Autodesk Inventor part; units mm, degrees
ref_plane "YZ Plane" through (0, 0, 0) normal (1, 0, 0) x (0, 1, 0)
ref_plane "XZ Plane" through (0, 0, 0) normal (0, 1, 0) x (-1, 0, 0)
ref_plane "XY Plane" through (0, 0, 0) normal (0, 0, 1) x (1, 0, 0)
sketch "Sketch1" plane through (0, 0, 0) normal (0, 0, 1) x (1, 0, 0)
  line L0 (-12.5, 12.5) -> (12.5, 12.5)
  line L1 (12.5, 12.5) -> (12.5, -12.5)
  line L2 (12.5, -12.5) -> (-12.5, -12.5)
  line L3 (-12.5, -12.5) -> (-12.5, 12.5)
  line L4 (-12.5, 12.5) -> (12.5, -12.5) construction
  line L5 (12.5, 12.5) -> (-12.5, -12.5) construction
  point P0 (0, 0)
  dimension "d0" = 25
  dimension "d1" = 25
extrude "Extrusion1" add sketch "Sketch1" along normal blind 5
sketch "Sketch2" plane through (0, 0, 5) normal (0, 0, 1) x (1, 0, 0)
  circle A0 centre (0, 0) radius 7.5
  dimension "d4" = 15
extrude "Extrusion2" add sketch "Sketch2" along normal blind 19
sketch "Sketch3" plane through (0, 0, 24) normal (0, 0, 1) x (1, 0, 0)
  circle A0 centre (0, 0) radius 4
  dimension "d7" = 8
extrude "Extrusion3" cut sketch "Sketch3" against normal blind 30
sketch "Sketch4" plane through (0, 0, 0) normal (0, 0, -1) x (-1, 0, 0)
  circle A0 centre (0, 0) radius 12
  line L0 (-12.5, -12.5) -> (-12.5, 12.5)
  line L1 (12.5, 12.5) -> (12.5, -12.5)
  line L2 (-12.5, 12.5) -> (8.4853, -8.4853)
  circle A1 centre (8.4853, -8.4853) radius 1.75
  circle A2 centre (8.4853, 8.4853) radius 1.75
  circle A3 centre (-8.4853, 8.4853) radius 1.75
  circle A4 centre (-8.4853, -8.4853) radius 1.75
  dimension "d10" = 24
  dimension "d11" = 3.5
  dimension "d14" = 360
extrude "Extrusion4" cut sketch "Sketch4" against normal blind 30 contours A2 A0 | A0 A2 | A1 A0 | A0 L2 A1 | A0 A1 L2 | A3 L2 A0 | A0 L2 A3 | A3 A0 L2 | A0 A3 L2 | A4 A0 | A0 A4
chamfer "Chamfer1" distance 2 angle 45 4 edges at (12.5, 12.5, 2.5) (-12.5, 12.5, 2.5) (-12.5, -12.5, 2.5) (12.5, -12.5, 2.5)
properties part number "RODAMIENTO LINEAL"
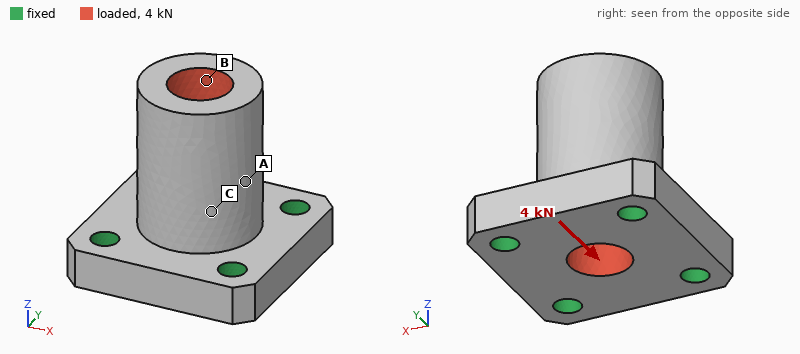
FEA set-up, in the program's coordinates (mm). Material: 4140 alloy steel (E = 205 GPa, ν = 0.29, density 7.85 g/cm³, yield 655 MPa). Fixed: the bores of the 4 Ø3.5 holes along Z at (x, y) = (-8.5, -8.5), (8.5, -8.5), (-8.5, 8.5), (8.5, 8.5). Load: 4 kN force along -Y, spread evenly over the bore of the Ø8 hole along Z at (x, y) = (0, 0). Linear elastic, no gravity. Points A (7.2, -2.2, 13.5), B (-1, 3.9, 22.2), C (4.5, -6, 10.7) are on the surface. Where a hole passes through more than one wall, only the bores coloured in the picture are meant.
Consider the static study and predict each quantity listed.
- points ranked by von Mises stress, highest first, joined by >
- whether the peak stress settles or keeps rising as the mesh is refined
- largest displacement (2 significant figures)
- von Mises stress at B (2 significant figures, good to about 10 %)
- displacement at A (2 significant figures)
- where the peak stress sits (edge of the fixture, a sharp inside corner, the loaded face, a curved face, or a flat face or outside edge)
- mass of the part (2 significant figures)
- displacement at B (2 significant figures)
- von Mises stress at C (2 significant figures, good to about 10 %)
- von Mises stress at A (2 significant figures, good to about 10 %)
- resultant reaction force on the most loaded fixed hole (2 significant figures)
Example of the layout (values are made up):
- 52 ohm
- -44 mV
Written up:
- C > A > B
- keeps rising
- 22 µm
- 13 MPa
- 10 µm
- edge of the fixture
- 40 g
- 20 µm
- 42 MPa
- 34 MPa
- 1.6 kN
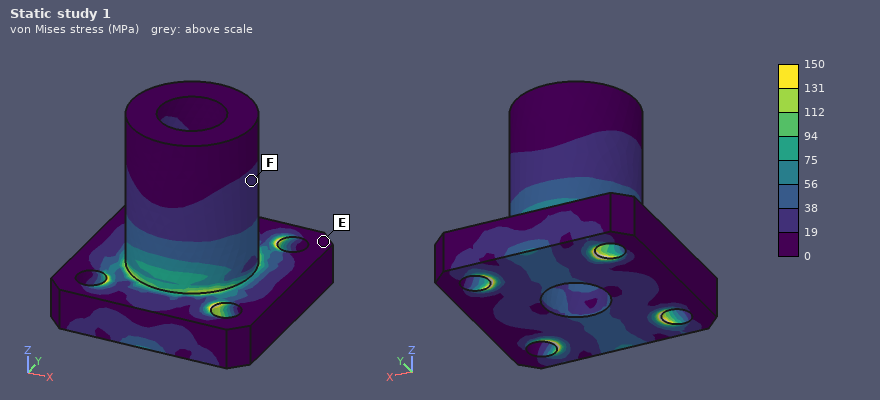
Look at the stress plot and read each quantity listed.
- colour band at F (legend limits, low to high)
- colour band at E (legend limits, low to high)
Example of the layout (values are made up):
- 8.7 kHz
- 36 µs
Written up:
- 19 to 38 MPa
- 0 to 19 MPa
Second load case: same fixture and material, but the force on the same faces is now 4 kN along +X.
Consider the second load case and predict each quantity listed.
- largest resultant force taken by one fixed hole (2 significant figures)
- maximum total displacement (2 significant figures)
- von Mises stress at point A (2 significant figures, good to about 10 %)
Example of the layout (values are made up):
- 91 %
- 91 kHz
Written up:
- 1.6 kN
- 22 µm
- 28 MPa
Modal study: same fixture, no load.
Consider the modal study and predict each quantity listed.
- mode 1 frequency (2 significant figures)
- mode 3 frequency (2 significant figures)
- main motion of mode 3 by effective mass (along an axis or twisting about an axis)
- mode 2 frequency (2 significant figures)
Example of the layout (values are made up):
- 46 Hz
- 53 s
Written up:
- 16 kHz
- 36 kHz
- along Z
- 16 kHz
